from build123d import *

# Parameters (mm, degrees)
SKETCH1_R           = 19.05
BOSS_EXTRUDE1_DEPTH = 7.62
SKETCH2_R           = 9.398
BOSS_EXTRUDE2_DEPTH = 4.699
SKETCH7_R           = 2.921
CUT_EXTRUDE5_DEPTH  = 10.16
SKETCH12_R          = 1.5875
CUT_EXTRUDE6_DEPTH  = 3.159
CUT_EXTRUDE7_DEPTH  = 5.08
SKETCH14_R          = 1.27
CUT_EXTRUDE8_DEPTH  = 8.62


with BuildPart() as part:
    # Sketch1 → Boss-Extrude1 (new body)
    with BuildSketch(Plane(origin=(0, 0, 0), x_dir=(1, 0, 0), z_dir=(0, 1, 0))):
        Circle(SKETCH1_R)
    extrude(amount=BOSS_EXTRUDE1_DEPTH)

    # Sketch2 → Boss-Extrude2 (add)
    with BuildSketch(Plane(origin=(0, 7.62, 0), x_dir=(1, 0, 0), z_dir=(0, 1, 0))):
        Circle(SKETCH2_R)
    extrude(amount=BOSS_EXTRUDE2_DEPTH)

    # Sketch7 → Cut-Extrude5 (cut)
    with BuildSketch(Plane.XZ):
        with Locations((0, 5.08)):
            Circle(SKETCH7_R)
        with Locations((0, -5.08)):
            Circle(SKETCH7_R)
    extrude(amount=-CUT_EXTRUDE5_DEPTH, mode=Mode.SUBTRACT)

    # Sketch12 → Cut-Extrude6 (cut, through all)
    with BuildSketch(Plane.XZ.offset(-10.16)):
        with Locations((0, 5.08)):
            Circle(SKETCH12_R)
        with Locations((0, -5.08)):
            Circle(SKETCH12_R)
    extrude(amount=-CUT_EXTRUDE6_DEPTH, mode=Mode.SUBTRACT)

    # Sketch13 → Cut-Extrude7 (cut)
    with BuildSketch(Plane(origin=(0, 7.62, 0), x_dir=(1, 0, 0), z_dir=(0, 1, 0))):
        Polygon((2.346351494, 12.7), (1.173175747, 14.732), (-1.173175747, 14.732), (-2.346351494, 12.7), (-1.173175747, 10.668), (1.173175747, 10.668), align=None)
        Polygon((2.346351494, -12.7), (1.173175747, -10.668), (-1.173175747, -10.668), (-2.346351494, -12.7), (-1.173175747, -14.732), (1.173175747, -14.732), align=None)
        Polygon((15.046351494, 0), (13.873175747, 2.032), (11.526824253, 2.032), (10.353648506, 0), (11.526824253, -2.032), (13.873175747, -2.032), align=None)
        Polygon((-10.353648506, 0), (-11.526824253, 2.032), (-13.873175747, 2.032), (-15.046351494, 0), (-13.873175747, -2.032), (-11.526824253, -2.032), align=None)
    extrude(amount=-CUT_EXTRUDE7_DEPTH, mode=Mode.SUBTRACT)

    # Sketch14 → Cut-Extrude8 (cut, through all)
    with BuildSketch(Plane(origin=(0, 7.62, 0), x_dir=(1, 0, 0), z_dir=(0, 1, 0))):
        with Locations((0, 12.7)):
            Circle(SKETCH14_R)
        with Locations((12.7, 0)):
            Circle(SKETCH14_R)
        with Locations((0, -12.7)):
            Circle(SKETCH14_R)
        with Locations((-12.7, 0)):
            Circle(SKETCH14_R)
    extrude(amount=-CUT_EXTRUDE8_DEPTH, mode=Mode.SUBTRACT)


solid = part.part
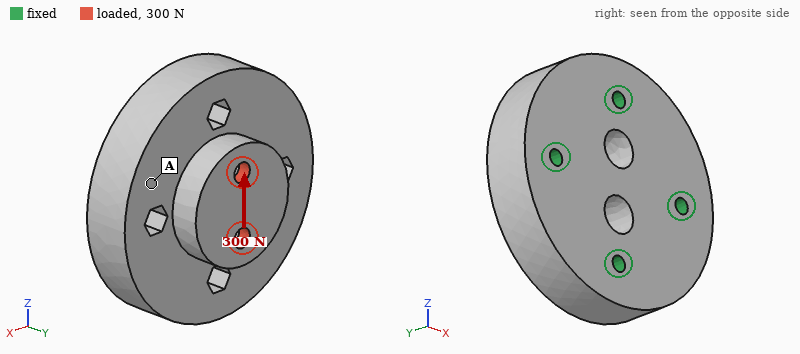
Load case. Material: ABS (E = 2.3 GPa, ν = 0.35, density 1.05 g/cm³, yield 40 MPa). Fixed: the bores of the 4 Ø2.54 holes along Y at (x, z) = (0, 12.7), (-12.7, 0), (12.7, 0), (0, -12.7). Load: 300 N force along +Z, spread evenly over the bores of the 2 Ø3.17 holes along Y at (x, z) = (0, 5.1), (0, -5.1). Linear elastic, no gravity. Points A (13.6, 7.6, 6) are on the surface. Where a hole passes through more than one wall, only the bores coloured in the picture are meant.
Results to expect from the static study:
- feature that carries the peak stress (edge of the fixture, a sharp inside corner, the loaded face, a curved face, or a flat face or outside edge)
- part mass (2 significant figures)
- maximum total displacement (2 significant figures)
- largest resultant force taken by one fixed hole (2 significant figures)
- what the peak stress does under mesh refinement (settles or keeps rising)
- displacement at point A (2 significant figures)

edge of the fixture
9.5 g
53 µm
140 N
keeps rising
16 µm
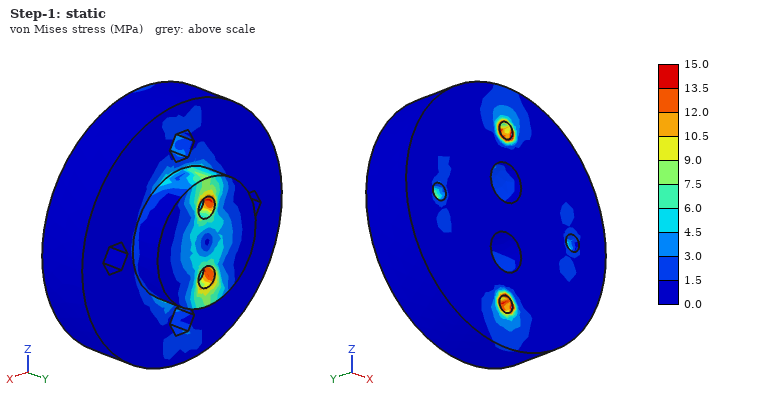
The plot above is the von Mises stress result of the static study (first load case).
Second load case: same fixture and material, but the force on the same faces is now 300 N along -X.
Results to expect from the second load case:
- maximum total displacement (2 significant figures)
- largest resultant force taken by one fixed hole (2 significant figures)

42 µm
150 N
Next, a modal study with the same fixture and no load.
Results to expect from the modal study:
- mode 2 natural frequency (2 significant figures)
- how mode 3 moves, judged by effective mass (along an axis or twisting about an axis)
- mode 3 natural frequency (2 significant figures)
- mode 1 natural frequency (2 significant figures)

7600 Hz
along Y
9400 Hz
7500 Hz
